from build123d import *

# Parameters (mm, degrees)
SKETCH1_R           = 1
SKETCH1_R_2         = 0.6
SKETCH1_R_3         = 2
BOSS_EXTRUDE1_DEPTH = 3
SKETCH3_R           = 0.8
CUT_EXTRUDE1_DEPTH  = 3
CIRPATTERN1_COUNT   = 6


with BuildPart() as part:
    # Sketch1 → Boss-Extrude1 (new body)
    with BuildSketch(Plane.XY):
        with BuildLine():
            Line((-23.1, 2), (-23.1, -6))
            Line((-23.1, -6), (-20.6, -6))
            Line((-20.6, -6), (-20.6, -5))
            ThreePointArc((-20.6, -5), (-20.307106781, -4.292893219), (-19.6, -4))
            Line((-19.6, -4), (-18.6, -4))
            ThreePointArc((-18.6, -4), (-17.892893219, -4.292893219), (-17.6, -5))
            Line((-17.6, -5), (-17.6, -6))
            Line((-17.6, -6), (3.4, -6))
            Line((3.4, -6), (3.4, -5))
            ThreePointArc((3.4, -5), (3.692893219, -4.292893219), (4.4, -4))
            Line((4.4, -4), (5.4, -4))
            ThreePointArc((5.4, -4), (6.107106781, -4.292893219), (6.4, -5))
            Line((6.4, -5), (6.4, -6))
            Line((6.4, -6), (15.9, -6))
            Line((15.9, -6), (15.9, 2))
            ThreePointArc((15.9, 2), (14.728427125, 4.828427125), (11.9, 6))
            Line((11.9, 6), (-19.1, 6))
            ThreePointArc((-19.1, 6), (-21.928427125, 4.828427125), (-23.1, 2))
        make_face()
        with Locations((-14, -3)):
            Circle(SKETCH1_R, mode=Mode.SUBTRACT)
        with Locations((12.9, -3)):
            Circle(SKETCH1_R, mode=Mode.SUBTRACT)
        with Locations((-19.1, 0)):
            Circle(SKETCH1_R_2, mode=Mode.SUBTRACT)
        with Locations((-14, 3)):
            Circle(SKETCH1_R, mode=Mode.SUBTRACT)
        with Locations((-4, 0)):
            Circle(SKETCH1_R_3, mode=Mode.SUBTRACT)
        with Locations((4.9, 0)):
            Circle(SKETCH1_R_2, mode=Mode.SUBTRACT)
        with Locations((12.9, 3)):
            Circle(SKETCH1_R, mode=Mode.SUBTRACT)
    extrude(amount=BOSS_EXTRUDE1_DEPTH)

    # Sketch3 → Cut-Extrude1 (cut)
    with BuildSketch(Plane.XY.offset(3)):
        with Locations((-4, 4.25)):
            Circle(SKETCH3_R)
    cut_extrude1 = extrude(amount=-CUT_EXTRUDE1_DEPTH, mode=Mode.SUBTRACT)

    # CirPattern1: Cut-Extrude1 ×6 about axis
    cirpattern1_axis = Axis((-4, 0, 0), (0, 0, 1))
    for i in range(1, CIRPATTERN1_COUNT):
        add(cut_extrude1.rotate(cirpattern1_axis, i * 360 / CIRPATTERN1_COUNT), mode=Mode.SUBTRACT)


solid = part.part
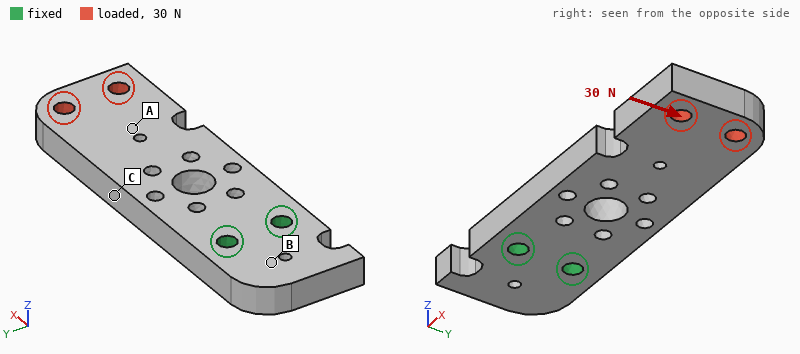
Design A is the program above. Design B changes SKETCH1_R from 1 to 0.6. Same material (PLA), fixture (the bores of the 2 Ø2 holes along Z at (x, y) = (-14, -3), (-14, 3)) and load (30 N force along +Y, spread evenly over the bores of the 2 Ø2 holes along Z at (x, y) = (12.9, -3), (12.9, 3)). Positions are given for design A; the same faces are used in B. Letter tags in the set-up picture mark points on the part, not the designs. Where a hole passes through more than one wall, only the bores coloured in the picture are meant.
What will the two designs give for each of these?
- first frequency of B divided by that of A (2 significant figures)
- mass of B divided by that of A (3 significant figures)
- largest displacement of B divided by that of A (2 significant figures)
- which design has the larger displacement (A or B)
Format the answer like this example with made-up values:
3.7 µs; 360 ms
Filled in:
0.94; 1.02; 1.1; B
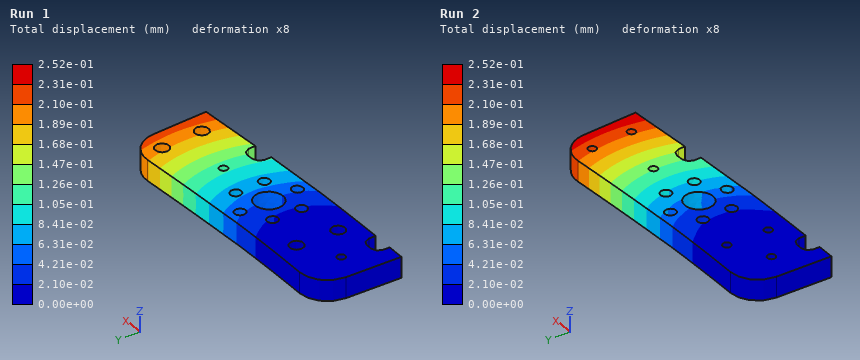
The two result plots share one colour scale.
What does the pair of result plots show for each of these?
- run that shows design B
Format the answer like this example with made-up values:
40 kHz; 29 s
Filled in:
Run 2
